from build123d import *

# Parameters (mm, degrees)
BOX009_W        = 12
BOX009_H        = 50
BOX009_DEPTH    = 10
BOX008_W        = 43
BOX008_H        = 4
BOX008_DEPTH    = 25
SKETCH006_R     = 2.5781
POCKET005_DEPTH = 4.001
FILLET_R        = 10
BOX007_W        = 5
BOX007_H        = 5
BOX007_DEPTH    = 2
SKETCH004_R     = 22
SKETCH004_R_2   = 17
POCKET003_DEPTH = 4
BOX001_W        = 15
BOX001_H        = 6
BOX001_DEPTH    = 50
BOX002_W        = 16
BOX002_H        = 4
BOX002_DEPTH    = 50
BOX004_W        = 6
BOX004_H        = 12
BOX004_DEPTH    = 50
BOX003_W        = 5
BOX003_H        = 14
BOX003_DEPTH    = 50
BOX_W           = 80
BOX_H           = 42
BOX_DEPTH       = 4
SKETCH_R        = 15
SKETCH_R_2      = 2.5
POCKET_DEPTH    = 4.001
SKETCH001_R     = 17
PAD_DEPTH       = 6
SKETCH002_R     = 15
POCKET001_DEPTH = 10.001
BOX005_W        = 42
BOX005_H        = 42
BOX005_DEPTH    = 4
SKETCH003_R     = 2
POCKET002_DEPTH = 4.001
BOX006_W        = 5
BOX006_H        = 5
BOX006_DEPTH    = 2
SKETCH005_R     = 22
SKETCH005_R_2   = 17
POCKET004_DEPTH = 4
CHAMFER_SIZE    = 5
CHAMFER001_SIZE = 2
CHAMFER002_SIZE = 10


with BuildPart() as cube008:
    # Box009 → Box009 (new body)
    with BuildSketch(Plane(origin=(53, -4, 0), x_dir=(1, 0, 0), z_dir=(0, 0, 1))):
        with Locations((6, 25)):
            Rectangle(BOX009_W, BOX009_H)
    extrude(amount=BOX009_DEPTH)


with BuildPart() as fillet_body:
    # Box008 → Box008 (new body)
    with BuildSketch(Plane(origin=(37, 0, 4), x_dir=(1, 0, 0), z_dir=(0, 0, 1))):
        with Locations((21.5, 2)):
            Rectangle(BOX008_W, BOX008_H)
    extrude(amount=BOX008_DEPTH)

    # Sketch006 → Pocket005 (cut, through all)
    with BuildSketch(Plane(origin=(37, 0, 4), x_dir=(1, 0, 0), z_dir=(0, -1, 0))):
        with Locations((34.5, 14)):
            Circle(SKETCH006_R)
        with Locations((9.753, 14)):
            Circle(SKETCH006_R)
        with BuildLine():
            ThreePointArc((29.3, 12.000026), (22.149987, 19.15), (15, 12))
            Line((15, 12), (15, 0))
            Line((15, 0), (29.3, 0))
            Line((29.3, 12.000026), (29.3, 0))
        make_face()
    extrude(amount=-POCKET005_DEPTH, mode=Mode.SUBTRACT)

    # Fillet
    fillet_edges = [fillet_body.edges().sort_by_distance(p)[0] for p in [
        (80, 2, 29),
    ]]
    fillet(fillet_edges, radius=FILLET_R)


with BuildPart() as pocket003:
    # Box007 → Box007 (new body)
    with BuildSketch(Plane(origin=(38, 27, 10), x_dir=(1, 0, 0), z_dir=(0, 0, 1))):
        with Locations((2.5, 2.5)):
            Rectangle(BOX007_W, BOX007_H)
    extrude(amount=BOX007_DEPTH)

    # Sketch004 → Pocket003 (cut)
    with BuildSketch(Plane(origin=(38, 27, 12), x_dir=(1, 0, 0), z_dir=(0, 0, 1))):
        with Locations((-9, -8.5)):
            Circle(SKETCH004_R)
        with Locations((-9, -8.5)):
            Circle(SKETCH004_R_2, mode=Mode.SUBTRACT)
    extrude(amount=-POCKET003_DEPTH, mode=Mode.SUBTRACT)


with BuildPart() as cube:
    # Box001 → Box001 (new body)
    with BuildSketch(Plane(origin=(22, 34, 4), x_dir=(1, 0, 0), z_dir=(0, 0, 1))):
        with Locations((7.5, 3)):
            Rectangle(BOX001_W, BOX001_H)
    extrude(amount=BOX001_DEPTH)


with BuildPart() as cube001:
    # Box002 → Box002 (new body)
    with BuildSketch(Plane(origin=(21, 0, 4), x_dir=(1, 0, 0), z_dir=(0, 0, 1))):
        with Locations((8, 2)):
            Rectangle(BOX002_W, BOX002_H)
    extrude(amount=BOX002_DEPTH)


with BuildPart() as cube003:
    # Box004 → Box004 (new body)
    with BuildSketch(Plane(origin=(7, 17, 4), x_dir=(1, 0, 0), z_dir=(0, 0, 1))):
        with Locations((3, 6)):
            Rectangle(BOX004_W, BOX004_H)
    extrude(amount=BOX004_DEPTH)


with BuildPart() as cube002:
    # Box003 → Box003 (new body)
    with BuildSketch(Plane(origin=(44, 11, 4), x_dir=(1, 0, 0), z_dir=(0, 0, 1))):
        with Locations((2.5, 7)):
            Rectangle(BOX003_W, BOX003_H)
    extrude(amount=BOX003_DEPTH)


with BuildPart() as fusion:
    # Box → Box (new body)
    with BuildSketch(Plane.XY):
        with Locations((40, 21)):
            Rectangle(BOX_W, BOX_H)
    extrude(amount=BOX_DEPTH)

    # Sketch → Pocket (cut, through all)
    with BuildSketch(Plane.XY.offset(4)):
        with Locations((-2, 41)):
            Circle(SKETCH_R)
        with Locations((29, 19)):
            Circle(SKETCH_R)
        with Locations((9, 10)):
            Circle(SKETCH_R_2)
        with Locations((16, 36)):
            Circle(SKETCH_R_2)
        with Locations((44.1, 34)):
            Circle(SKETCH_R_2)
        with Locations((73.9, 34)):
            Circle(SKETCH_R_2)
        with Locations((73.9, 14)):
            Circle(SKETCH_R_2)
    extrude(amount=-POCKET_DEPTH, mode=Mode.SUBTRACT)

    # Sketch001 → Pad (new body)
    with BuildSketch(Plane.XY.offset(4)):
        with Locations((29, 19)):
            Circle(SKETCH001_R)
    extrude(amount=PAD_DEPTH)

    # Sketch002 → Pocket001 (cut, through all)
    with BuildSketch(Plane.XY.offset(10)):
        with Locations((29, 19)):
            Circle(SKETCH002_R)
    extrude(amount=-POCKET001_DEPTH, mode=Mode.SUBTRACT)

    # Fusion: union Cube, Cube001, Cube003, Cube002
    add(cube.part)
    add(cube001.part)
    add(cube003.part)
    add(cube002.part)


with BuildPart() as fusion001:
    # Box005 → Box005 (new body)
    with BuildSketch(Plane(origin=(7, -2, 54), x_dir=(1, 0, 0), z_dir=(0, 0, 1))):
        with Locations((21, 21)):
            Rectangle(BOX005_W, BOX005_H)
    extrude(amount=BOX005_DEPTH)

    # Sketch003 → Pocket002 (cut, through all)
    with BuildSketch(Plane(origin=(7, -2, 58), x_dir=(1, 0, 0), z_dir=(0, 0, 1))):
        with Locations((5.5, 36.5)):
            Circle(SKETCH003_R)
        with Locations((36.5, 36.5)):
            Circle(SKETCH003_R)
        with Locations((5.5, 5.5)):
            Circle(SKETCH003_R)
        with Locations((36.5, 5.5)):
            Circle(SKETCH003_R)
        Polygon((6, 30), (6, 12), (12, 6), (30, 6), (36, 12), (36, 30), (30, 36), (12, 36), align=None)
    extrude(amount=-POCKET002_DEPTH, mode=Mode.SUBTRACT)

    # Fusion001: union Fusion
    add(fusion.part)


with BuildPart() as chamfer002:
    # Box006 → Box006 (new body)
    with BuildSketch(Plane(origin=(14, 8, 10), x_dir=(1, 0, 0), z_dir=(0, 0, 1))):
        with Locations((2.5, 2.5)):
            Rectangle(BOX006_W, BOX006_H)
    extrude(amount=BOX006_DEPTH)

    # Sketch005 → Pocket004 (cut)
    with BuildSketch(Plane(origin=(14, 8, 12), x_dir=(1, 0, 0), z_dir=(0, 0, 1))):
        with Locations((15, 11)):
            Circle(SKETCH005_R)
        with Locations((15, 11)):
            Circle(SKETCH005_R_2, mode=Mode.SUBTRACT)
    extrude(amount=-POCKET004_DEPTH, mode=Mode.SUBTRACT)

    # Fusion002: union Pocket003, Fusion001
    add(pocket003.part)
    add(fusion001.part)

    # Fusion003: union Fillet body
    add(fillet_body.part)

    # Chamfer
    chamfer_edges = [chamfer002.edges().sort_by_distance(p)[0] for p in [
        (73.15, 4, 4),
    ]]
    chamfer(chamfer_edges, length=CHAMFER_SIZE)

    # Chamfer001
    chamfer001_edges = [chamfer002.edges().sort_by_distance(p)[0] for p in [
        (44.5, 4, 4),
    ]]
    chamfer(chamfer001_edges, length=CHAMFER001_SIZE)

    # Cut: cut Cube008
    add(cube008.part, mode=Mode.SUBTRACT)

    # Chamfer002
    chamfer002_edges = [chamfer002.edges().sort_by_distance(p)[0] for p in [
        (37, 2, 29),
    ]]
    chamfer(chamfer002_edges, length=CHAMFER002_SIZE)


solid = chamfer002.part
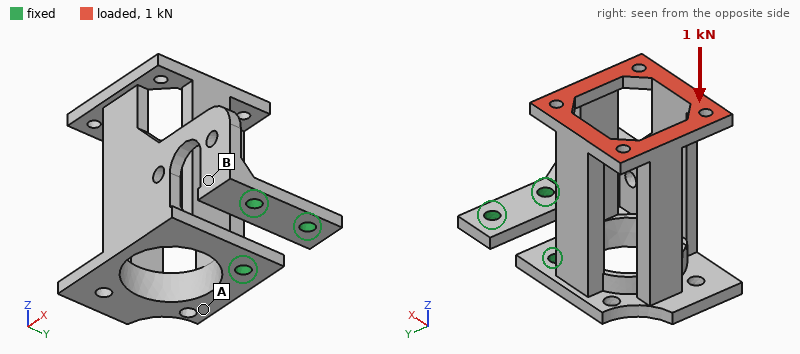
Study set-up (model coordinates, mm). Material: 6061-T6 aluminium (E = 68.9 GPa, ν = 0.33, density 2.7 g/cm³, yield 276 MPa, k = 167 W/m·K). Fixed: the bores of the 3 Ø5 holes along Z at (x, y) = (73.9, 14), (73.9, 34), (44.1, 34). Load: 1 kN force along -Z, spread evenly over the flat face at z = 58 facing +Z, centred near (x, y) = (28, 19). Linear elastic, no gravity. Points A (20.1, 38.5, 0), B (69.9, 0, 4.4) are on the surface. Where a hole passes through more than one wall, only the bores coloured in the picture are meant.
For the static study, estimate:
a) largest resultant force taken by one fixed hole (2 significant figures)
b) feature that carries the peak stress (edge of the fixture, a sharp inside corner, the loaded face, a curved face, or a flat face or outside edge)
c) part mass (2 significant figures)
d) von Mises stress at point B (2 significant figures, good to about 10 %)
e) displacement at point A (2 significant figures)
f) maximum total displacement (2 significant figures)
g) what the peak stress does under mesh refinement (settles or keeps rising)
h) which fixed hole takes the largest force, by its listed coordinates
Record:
980 N
edge of the fixture
82 g
42 MPa
0.15 mm
0.92 mm
keeps rising
(44.1, 34)
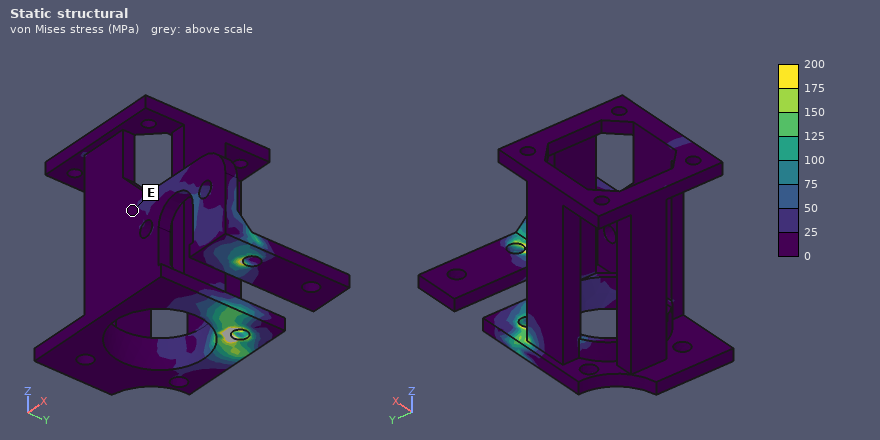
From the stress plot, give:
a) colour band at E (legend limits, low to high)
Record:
0 to 25 MPa
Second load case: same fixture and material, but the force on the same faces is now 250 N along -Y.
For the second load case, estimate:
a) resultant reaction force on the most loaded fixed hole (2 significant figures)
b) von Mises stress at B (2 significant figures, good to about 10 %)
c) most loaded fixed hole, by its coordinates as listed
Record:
300 N
25 MPa
(44.1, 34)
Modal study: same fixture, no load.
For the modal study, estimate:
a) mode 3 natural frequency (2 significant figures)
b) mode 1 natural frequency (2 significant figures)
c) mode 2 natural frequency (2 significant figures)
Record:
1900 Hz
620 Hz
1500 Hz
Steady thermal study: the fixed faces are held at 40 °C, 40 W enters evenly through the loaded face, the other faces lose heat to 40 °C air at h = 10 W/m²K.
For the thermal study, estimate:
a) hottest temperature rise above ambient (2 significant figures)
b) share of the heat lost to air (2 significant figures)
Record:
75 K
16 %
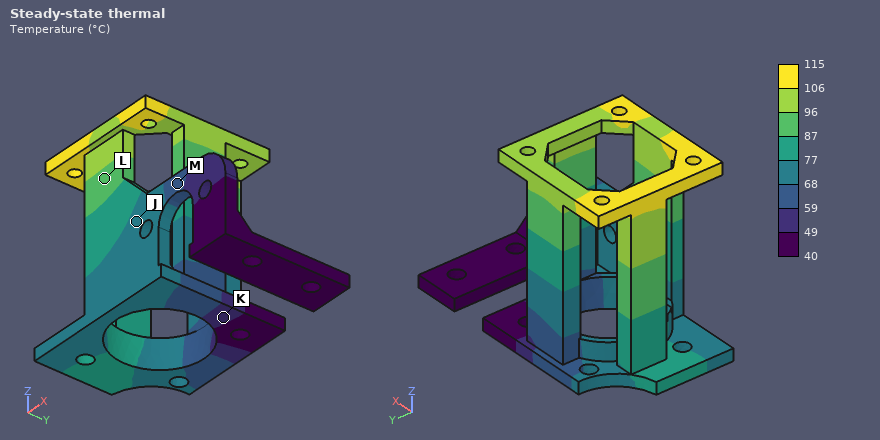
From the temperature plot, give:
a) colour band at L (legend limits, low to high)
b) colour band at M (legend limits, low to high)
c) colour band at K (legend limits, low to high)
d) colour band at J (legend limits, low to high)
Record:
87 to 96 °C
59 to 68 °C
49 to 59 °C
68 to 77 °C
